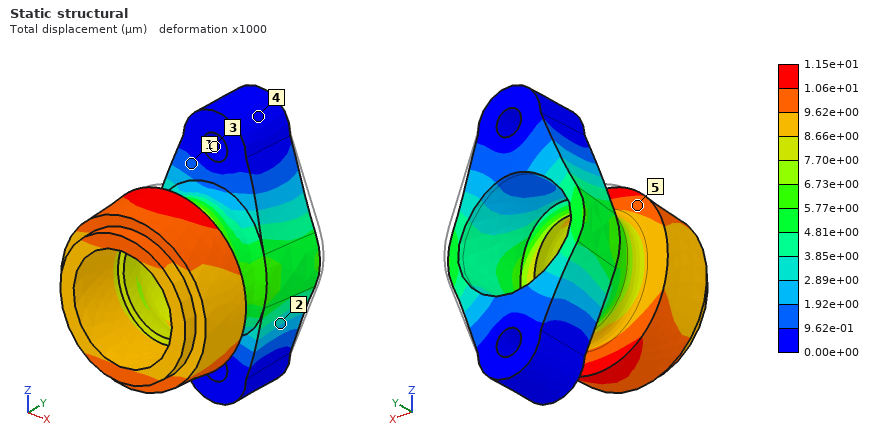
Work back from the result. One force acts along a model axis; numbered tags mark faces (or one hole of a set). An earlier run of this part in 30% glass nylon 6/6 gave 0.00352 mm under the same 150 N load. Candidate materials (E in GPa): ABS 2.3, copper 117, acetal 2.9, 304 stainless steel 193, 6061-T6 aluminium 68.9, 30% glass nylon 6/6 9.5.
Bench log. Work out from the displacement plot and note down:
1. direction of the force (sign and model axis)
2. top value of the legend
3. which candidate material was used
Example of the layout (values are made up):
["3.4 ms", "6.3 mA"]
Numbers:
["-Y", "1.15e+01 µm", "acetal"]
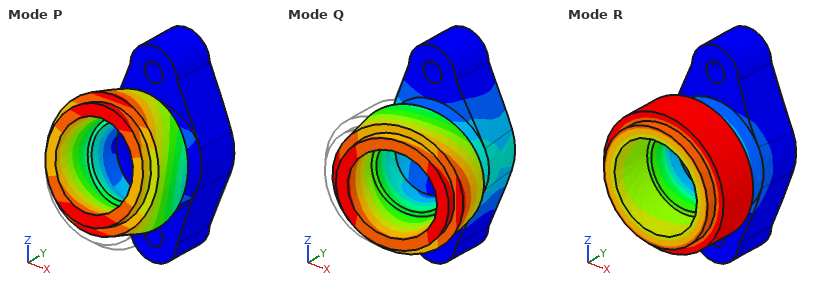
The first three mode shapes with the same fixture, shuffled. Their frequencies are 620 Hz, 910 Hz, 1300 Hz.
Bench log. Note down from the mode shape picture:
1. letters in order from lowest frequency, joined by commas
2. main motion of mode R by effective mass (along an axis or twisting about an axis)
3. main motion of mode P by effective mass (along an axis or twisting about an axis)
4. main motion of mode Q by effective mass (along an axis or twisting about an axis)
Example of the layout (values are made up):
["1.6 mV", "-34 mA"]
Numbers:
["Q, P, R", "twisting about Y", "along Z", "along X"]
